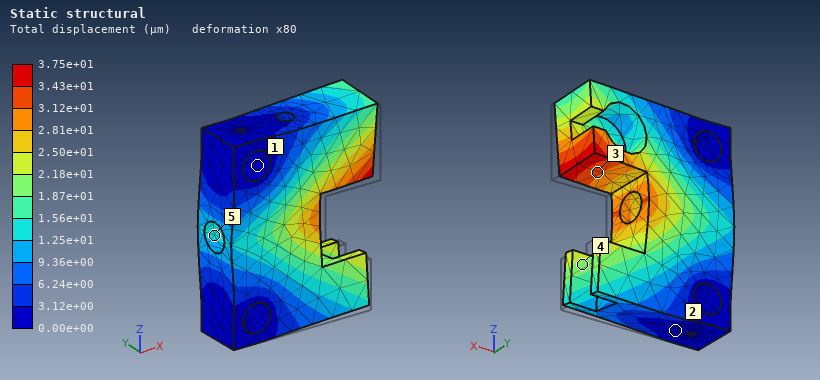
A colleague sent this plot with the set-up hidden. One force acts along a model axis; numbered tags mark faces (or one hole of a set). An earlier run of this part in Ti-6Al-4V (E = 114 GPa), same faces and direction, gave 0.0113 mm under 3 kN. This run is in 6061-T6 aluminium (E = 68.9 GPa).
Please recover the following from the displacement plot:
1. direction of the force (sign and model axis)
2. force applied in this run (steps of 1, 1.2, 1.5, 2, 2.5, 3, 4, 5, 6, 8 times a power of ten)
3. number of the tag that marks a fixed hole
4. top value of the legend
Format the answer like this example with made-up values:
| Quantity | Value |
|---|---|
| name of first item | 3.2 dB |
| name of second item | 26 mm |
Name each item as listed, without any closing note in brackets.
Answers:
| Quantity | Value |
|---|---|
| direction of the force | +Y |
| force applied in this run | 6 kN |
| number of the tag that marks a fixed hole | 1 |
| top value of the legend | 3.75e+01 µm |
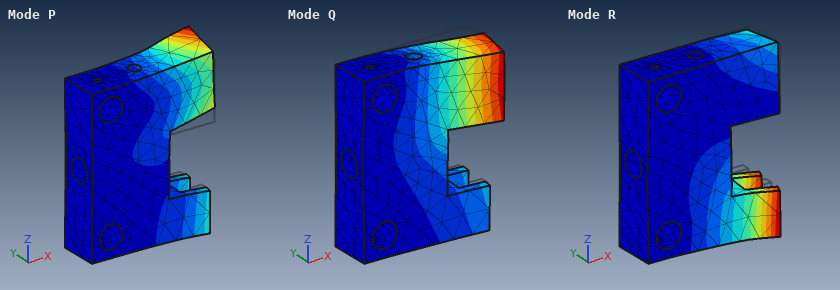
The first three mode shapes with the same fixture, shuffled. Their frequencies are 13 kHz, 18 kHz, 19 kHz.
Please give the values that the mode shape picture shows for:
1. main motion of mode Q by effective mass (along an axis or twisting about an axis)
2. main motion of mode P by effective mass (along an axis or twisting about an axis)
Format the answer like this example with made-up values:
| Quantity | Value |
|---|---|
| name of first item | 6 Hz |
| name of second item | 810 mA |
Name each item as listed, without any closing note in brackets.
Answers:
| Quantity | Value |
|---|---|
| main motion of mode Q by effective mass | along Y |
| main motion of mode P by effective mass | along Z |
